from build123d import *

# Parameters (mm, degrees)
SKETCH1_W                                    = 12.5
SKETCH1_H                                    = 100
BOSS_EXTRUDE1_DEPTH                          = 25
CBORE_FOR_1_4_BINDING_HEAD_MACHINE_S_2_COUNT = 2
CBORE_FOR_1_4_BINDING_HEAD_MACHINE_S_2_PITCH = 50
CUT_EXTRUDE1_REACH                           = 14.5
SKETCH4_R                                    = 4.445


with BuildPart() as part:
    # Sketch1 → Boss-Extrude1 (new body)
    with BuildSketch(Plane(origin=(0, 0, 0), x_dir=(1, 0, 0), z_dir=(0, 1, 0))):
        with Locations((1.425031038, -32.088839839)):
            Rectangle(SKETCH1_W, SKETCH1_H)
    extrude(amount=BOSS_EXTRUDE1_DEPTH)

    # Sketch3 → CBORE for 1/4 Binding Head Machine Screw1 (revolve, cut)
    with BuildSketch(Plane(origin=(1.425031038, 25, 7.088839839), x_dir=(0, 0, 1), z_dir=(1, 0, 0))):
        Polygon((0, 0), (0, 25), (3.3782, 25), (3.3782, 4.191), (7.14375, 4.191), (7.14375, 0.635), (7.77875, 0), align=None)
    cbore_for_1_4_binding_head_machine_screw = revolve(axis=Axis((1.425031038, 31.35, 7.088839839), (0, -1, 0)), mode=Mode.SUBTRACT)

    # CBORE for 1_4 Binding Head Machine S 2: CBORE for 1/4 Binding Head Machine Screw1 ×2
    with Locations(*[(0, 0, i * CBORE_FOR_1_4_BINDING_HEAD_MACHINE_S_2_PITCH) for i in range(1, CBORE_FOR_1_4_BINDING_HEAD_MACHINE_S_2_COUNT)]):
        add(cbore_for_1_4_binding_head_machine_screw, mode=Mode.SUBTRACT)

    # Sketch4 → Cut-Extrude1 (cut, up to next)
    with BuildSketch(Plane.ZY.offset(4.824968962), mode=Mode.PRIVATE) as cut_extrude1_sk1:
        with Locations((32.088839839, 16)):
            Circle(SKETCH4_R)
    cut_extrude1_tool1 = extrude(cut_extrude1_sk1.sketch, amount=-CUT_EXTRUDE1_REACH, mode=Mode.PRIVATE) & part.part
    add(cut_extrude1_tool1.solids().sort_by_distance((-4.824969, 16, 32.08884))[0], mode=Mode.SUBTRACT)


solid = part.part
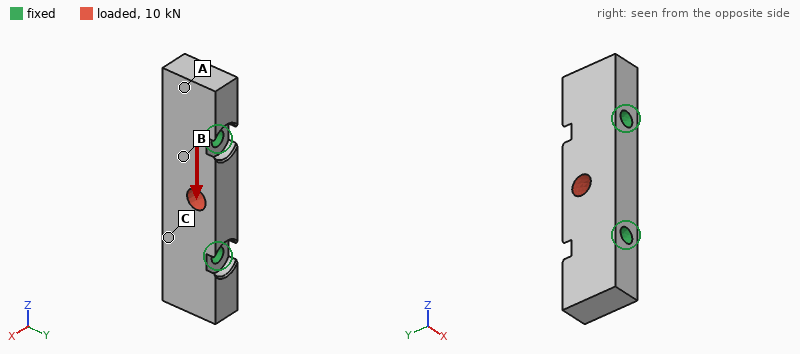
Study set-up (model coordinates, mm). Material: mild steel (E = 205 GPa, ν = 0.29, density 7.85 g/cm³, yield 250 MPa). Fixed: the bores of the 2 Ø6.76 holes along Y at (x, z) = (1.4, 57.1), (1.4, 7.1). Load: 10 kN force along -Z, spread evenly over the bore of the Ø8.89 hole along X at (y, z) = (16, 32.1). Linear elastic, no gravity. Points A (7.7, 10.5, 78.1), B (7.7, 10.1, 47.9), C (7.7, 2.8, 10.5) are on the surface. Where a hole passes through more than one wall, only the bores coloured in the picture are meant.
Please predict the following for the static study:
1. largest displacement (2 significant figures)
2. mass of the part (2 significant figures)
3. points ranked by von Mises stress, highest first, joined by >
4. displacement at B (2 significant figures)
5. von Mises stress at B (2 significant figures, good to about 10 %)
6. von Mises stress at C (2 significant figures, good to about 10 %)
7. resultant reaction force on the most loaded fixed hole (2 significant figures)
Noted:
3.1 µm
220 g
B > C > A
0.65 µm
16 MPa
7.8 MPa
5.1 kN
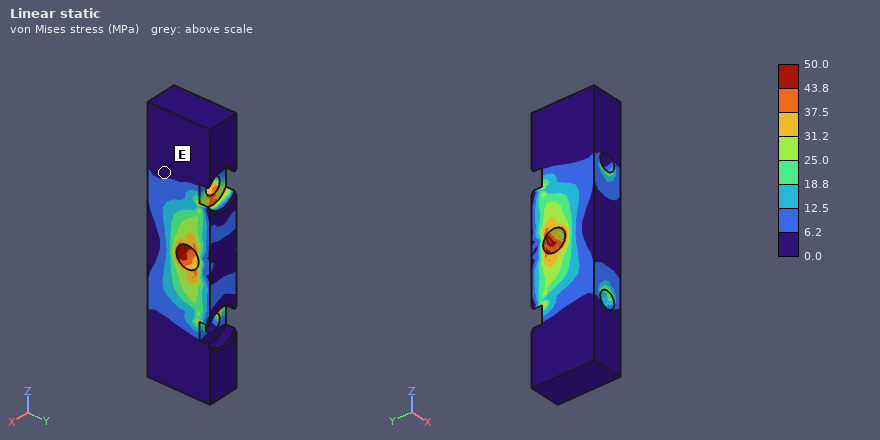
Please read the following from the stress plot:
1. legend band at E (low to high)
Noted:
0.0 to 6.2 MPa
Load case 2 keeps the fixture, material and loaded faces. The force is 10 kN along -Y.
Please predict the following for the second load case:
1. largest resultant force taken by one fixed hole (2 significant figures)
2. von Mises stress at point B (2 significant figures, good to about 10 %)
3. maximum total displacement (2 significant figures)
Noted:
5.1 kN
44 MPa
8.5 µm
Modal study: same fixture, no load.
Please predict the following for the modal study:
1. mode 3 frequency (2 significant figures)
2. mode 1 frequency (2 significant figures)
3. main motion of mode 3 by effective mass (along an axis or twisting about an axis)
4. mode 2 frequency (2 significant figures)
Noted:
20 kHz
13 kHz
along X
13 kHz
